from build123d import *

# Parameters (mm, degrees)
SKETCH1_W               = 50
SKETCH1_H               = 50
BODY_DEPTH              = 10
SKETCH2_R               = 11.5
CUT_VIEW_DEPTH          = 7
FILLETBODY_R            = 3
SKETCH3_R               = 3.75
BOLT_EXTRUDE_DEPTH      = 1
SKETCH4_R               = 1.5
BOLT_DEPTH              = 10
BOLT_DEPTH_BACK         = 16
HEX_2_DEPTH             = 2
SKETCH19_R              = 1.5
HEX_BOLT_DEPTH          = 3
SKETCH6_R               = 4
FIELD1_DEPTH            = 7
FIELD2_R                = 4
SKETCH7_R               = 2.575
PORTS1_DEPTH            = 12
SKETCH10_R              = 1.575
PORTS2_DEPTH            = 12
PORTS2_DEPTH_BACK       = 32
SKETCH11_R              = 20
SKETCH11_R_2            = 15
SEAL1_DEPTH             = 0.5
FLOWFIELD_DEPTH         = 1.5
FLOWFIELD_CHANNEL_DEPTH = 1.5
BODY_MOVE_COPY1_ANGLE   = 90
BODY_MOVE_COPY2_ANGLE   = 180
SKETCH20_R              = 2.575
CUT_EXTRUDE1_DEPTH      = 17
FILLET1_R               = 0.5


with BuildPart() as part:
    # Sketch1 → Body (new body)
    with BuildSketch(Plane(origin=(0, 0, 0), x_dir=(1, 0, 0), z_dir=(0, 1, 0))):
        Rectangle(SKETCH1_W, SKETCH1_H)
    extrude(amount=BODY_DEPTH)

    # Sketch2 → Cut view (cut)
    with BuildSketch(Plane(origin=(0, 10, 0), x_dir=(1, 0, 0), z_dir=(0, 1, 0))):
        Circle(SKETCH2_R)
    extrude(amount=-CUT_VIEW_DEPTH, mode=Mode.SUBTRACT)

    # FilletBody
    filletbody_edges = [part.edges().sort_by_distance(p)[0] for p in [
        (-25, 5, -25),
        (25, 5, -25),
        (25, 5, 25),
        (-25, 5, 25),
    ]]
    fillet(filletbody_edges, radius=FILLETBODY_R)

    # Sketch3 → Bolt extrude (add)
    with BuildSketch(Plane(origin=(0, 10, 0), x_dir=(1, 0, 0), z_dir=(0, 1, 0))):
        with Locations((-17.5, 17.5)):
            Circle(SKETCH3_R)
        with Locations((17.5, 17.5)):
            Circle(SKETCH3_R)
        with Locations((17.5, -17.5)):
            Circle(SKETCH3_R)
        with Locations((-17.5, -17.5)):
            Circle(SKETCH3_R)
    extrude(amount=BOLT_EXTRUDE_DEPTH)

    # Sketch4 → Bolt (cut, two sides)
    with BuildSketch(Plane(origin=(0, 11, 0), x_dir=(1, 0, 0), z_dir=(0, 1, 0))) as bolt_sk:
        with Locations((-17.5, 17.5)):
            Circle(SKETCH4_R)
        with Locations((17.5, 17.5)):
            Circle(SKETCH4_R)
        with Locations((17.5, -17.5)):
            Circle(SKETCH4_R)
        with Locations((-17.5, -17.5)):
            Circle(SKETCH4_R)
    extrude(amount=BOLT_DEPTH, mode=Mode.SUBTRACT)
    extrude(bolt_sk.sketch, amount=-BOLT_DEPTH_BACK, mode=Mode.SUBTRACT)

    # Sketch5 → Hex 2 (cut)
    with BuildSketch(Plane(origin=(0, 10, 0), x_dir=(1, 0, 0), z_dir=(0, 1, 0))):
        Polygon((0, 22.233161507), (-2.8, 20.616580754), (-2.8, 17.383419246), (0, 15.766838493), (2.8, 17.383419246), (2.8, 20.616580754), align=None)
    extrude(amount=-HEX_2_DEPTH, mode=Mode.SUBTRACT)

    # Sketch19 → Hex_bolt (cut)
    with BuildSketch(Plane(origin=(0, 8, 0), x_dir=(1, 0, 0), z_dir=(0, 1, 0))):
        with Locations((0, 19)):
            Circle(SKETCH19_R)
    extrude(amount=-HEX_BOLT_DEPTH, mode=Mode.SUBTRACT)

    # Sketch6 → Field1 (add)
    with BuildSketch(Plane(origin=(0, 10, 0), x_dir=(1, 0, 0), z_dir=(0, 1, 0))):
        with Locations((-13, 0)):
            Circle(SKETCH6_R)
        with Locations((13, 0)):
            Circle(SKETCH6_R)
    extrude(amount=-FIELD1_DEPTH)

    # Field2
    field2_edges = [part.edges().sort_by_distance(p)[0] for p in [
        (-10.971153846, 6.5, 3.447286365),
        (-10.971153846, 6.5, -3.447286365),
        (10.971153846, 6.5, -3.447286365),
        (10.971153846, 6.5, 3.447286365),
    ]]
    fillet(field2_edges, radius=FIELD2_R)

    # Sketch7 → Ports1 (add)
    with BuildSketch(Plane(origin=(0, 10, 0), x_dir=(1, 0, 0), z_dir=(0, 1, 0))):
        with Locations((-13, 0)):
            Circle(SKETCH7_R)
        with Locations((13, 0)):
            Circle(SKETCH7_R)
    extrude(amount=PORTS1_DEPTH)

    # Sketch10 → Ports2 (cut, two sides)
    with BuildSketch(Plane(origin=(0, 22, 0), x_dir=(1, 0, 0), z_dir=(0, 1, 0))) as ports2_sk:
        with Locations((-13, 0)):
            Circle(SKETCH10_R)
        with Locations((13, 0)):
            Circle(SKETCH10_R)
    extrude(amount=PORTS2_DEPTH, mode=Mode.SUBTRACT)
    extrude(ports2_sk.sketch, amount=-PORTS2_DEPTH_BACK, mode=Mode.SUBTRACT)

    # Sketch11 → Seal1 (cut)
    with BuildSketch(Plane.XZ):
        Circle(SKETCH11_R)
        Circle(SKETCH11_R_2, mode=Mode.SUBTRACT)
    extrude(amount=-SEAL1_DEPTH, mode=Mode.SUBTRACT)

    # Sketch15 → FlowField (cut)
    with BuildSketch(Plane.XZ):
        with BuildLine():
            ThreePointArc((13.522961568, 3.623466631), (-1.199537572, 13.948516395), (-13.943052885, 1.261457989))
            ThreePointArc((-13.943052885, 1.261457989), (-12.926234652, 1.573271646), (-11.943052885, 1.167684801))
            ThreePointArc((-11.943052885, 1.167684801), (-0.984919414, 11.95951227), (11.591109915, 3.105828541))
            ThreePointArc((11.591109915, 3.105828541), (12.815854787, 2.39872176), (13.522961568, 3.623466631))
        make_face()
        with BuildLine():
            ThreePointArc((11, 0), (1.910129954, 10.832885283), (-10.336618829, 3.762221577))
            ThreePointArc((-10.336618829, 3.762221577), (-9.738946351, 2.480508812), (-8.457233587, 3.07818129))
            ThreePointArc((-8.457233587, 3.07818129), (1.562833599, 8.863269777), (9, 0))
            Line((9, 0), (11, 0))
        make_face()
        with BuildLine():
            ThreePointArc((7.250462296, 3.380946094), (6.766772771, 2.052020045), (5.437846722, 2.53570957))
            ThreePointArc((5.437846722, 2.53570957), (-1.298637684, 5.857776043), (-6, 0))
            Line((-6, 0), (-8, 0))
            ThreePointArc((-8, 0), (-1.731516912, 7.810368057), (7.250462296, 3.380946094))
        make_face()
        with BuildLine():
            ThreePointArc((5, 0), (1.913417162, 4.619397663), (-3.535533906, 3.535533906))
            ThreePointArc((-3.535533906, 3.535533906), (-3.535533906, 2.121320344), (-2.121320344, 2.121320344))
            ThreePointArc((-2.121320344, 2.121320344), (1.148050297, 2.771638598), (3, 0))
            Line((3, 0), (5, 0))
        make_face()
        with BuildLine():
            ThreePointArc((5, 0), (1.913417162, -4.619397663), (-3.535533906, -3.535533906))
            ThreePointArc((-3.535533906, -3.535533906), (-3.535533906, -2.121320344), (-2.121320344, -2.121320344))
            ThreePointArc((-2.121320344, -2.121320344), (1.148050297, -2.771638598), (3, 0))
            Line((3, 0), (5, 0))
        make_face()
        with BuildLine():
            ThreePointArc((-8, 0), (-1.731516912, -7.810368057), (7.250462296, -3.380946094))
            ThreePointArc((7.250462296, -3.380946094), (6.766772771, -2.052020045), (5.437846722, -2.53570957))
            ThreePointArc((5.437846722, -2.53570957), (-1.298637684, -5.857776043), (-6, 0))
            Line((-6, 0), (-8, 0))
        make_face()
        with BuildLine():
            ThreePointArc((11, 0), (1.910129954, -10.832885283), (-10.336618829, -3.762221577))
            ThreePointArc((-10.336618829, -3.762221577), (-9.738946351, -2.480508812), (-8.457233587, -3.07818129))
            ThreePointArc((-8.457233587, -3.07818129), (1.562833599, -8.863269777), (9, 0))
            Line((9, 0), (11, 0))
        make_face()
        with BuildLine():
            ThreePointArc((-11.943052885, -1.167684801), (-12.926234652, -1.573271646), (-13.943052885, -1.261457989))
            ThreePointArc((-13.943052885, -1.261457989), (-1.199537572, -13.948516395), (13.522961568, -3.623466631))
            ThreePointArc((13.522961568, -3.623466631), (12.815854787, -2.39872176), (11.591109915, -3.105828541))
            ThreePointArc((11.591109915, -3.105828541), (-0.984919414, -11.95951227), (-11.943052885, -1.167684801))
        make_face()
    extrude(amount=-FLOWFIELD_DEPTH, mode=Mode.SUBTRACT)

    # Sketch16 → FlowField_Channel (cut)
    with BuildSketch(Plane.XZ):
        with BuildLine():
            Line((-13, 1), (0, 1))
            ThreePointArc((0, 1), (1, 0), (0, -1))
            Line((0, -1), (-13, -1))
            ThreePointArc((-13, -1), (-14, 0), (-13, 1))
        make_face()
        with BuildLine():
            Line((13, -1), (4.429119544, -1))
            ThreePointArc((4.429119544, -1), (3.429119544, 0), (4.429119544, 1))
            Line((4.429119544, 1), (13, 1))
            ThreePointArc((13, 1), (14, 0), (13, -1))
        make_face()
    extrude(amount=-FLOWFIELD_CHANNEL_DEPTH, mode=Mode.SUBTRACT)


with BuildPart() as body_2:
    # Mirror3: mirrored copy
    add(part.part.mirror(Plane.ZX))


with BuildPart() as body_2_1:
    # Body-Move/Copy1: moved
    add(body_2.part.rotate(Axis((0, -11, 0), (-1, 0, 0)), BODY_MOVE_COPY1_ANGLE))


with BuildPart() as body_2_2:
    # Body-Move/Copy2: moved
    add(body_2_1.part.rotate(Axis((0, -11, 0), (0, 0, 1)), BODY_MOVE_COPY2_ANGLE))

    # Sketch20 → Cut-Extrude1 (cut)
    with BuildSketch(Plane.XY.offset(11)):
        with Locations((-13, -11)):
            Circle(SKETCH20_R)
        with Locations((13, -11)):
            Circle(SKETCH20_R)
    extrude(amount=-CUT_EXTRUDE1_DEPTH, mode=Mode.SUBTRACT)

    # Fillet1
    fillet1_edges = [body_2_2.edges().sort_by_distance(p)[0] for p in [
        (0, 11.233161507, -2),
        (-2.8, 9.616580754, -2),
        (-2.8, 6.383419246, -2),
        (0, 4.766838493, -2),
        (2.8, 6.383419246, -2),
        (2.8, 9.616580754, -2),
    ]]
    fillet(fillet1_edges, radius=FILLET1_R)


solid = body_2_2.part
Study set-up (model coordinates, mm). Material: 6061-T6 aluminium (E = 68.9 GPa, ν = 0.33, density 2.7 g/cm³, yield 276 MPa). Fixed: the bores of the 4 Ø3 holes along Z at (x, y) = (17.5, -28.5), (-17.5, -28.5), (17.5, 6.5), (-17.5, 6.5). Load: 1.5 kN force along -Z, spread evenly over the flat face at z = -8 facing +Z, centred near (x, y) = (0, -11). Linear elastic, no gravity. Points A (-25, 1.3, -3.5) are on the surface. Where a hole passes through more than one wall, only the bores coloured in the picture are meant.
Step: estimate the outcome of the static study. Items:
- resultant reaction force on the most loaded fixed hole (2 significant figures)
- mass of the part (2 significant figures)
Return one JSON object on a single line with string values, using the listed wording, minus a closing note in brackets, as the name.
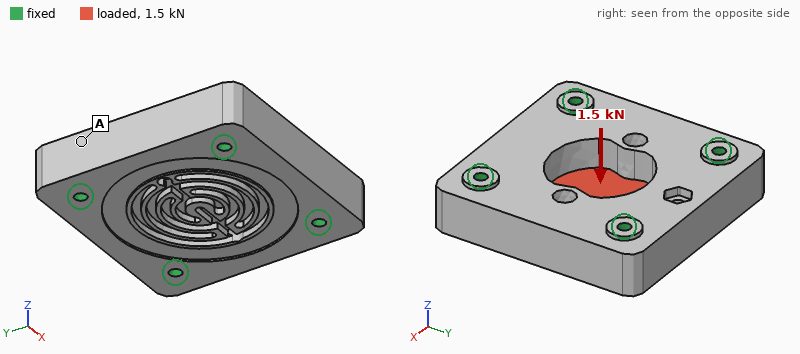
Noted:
{"resultant reaction force on the most loaded fixed hole": "430 N", "mass of the part": "56 g"}
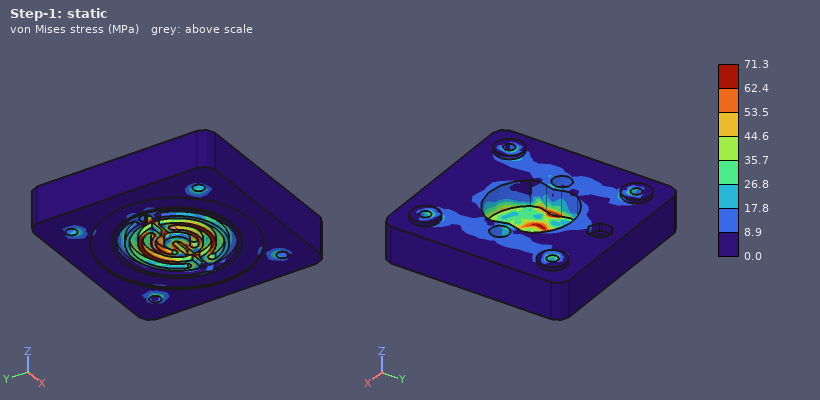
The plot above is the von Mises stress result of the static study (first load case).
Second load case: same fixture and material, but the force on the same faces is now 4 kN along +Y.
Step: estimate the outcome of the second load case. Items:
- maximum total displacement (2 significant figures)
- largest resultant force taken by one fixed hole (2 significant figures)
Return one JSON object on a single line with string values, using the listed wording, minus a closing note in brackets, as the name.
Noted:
{"maximum total displacement": "9.7 µm", "largest resultant force taken by one fixed hole": "1.1 kN"}
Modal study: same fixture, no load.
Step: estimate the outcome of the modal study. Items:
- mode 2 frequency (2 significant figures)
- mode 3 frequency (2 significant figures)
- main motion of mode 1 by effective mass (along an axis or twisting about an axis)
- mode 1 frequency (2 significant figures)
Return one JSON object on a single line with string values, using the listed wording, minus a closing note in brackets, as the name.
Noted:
{"mode 2 frequency": "28 kHz", "mode 3 frequency": "28 kHz", "main motion of mode 1 by effective mass": "along Z", "mode 1 frequency": "23 kHz"}
